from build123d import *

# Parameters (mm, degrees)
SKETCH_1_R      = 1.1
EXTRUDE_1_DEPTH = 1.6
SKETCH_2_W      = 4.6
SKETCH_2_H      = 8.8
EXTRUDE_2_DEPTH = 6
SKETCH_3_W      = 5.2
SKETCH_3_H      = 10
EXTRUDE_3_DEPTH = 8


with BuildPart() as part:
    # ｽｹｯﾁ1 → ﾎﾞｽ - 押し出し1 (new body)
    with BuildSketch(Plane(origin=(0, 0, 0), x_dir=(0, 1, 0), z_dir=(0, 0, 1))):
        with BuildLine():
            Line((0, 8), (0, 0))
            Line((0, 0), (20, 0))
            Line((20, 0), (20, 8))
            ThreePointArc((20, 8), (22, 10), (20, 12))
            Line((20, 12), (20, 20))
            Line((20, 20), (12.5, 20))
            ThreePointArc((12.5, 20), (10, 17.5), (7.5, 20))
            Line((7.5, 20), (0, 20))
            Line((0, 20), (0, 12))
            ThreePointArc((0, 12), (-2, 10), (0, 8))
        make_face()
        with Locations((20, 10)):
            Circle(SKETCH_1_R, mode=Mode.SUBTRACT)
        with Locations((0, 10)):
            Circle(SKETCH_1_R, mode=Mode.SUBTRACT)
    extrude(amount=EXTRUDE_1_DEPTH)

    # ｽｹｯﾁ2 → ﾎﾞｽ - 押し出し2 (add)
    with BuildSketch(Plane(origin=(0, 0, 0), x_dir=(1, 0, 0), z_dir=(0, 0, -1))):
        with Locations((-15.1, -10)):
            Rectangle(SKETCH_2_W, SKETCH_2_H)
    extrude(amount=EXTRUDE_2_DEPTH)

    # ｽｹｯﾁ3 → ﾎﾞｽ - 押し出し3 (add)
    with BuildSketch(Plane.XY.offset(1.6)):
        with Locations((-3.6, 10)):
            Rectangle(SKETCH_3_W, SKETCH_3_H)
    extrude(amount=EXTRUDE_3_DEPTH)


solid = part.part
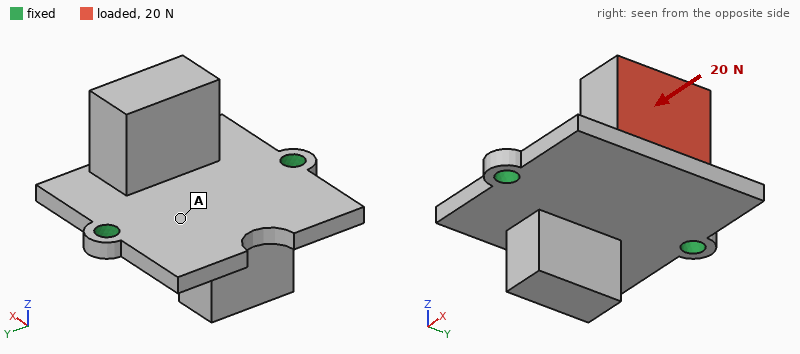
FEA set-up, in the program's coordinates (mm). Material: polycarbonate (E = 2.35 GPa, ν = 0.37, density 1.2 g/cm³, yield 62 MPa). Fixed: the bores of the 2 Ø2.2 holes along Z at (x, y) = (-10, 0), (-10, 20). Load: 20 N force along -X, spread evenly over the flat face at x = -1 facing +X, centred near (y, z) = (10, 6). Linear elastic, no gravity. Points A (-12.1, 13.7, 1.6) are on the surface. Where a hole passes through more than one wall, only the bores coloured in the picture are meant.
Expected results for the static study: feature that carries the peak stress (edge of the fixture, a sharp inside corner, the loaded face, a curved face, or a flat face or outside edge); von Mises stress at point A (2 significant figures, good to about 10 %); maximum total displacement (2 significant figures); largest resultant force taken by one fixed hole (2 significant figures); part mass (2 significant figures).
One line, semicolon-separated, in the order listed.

a flat face or outside edge; 2.8 MPa; 0.41 mm; 10 N; 1.5 g
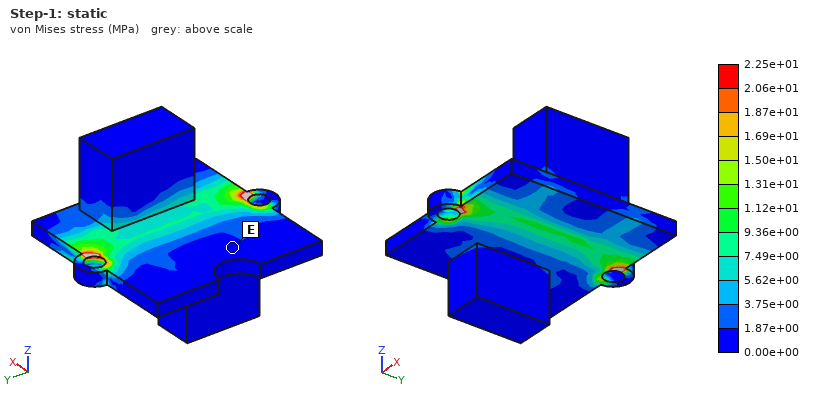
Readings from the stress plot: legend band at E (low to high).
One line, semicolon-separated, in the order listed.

0.00e+00 to 1.87e+00 MPa
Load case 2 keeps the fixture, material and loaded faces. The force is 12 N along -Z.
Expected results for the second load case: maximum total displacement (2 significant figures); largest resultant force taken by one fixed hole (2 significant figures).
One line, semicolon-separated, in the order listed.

0.38 mm; 6.3 N
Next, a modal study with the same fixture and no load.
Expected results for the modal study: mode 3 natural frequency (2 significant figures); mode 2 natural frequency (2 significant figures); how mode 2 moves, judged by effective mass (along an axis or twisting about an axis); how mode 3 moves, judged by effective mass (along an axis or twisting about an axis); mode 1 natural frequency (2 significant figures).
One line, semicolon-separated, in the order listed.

4100 Hz; 2300 Hz; along Z; along Y; 1300 Hz
